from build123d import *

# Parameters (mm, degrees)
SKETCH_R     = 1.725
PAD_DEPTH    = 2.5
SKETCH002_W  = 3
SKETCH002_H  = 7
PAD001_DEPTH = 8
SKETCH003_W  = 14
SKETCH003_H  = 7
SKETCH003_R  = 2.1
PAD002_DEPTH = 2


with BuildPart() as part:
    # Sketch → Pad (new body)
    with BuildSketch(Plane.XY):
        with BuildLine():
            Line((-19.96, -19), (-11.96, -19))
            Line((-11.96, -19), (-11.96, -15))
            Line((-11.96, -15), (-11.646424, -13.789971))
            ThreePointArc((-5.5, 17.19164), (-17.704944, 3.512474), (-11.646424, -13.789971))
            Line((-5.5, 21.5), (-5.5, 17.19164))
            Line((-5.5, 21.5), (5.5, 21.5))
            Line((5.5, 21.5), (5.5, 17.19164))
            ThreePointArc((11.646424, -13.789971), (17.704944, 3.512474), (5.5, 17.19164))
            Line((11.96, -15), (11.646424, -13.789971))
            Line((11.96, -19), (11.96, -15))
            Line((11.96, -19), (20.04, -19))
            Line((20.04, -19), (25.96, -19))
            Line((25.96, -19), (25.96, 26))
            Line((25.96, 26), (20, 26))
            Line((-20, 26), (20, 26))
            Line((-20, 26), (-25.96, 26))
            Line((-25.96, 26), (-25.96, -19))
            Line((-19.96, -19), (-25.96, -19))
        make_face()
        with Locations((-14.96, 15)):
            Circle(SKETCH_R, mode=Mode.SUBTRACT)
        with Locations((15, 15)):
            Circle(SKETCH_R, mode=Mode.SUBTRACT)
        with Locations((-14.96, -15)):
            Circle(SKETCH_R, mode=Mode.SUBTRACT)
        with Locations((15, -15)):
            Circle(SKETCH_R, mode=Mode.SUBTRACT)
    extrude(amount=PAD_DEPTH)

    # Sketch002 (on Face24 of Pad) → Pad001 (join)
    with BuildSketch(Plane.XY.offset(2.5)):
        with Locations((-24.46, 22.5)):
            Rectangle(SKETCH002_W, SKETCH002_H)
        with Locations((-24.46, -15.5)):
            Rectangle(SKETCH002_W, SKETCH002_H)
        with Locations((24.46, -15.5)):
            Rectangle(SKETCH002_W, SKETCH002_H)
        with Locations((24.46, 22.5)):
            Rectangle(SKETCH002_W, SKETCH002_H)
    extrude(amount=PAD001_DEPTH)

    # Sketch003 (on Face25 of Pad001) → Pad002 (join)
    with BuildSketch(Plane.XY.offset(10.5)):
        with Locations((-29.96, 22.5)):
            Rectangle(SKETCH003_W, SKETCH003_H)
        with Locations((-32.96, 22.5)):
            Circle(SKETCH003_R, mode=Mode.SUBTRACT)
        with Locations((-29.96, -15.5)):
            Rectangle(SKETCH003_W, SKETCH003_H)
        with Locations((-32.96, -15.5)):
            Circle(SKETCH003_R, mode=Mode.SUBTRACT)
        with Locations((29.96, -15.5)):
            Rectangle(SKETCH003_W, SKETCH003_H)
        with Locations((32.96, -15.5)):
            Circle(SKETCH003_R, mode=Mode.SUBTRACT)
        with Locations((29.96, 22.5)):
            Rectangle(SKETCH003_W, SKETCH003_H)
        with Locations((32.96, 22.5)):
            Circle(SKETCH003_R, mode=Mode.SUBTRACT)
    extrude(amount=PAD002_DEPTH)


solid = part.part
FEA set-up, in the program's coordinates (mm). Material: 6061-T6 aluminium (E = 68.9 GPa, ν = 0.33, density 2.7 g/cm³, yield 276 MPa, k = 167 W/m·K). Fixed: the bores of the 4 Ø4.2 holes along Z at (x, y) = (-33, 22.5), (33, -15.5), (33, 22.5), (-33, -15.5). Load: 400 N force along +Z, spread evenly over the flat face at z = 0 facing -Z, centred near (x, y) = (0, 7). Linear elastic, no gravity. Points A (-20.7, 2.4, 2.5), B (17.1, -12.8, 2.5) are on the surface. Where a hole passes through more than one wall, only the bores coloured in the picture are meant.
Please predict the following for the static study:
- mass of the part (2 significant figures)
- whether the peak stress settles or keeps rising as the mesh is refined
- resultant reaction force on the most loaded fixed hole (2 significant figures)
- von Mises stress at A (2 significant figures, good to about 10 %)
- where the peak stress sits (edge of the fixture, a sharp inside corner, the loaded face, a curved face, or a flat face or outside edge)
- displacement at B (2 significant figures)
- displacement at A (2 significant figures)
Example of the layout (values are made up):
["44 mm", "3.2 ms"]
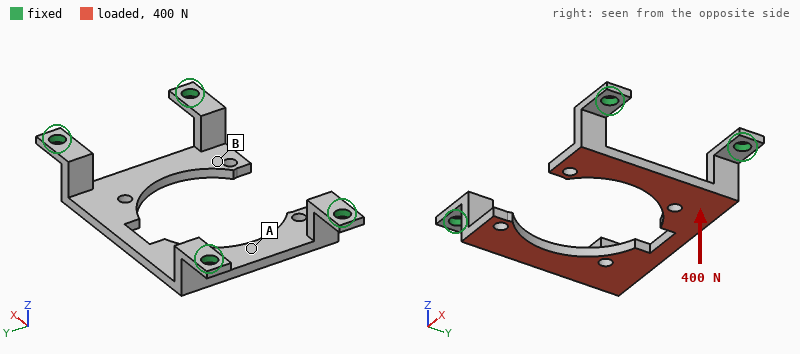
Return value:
["12 g", "keeps rising", "180 N", "22 MPa", "edge of the fixture", "0.11 mm", "0.073 mm"]
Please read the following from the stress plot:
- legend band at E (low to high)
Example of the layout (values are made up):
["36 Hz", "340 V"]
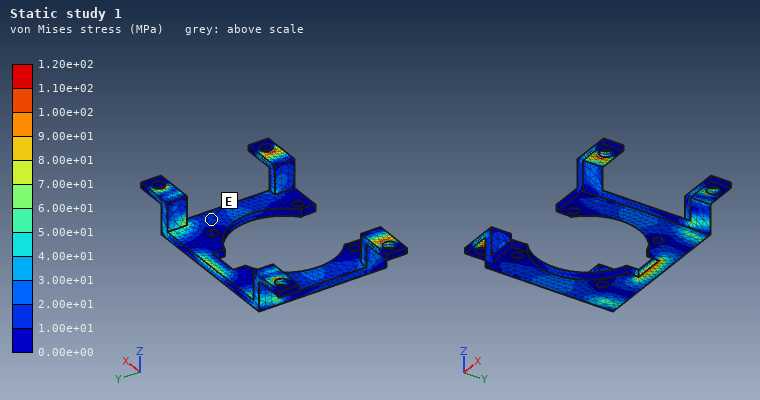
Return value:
["1.00e+01 to 2.00e+01 MPa"]
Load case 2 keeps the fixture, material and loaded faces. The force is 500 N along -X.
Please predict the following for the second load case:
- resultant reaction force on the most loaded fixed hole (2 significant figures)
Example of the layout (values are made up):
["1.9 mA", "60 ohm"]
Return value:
["190 N"]
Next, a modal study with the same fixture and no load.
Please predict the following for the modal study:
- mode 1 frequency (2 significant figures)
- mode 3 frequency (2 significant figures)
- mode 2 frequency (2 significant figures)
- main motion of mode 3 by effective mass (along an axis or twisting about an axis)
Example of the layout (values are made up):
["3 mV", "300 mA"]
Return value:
["2900 Hz", "4700 Hz", "3000 Hz", "along Y"]
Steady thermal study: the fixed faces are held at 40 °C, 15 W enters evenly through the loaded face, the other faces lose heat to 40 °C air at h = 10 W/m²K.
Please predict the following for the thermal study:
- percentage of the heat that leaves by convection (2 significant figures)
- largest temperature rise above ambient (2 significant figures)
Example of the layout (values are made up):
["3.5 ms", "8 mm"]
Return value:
["3.9 %", "29 K"]
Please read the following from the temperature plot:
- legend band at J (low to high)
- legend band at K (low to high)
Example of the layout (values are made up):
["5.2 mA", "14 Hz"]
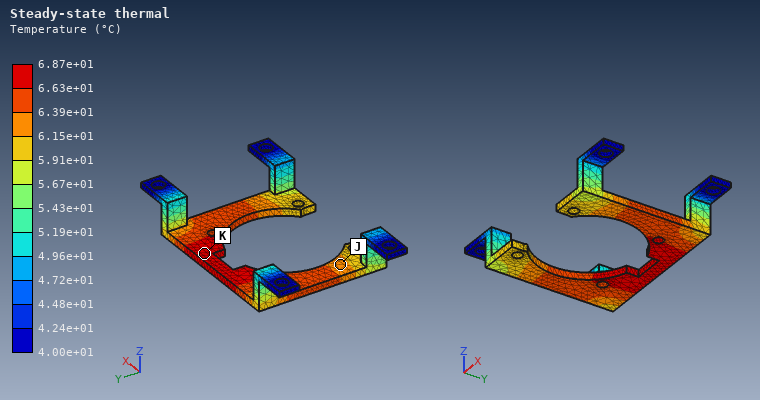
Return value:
["6.15e+01 to 6.39e+01 °C", "6.63e+01 to 6.87e+01 °C"]
